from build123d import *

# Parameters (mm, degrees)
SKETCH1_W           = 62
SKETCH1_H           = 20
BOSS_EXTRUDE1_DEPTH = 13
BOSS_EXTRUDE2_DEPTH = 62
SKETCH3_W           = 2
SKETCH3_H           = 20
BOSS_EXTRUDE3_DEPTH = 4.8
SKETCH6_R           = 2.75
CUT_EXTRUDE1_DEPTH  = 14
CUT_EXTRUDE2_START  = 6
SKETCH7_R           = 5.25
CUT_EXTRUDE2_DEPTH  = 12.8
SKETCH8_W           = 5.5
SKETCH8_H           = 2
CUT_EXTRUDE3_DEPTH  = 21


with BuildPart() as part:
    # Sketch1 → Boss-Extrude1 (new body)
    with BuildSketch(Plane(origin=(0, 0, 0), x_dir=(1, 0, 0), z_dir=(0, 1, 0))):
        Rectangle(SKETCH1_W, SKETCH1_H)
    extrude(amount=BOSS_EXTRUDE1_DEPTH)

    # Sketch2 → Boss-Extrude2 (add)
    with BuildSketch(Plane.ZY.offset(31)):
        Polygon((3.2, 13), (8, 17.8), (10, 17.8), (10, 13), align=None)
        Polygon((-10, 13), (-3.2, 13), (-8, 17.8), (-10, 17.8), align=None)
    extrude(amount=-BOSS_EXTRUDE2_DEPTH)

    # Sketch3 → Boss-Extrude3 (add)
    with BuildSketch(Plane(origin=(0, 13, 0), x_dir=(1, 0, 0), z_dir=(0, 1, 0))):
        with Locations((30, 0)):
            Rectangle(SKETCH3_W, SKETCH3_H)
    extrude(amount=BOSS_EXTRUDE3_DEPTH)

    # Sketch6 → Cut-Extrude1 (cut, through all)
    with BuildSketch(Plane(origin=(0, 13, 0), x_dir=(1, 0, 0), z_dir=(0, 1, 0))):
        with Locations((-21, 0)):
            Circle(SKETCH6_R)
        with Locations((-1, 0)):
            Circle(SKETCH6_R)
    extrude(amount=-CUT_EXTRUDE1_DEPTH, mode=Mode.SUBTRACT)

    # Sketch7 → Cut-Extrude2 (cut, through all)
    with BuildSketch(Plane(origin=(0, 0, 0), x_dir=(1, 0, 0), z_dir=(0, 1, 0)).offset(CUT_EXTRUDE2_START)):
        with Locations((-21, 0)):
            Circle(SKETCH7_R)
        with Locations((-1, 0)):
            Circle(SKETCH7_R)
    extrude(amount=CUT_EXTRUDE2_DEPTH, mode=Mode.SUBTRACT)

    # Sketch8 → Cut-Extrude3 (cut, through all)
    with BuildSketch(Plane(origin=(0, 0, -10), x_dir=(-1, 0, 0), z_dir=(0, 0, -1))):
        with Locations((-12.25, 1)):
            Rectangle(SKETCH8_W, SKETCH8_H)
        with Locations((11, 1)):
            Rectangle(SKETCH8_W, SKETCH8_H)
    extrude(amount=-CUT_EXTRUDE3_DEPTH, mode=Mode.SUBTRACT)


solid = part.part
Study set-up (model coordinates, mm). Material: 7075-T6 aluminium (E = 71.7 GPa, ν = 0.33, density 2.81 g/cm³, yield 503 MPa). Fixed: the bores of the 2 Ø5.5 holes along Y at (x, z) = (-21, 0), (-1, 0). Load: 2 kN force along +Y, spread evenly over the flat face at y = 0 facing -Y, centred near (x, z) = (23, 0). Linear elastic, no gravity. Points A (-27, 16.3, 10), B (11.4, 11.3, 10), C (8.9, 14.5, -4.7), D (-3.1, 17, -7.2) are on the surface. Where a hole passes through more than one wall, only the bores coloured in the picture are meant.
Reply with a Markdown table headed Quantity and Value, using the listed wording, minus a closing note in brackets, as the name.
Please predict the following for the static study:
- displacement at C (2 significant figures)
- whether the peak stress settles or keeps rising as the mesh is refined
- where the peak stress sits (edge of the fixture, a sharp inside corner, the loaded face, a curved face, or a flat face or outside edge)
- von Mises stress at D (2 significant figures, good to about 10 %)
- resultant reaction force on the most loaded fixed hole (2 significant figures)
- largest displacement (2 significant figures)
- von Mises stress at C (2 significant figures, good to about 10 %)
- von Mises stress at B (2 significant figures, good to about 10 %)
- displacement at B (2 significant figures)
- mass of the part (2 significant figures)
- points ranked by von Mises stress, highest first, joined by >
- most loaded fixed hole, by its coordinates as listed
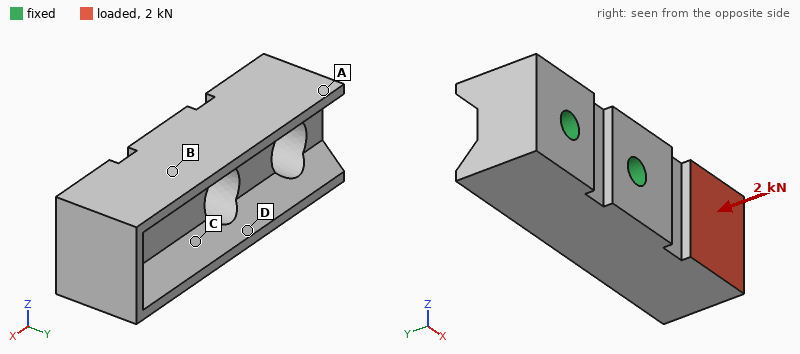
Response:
| Quantity | Value |
|---|---|
| displacement at C | 26 µm |
| whether the peak stress settles or keeps rising as the mesh is refined | keeps rising |
| where the peak stress sits | edge of the fixture |
| von Mises stress at D | 54 MPa |
| resultant reaction force on the most loaded fixed hole | 3.9 kN |
| largest displacement | 81 µm |
| von Mises stress at C | 37 MPa |
| von Mises stress at B | 25 MPa |
| displacement at B | 27 µm |
| mass of the part | 47 g |
| points ranked by von Mises stress, highest first, joined by > | D > C > B > A |
| most loaded fixed hole, by its coordinates as listed | (-1, 0) |
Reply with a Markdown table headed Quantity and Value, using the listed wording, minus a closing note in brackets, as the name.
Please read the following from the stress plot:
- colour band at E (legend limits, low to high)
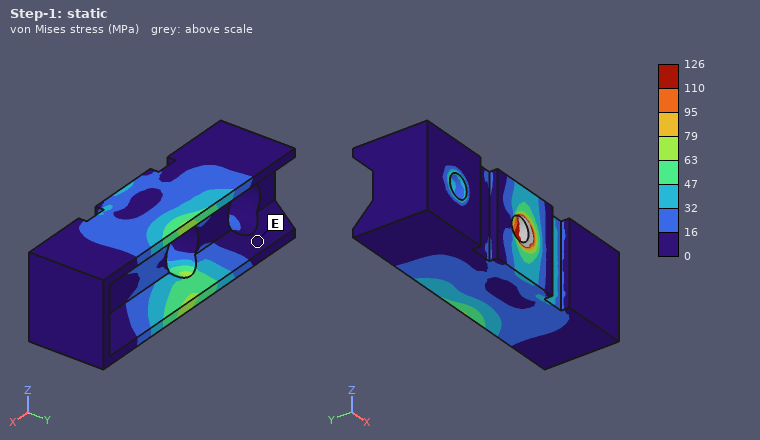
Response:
| Quantity | Value |
|---|---|
| colour band at E | 0 to 16 MPa |
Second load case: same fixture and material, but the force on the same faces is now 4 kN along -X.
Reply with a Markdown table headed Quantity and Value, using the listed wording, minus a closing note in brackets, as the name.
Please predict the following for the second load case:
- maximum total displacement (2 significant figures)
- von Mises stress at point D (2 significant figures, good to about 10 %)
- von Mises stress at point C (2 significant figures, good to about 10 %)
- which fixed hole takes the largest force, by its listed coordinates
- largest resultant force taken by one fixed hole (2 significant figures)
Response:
| Quantity | Value |
|---|---|
| maximum total displacement | 56 µm |
| von Mises stress at point D | 19 MPa |
| von Mises stress at point C | 27 MPa |
| which fixed hole takes the largest force, by its listed coordinates | (-1, 0) |
| largest resultant force taken by one fixed hole | 3.9 kN |
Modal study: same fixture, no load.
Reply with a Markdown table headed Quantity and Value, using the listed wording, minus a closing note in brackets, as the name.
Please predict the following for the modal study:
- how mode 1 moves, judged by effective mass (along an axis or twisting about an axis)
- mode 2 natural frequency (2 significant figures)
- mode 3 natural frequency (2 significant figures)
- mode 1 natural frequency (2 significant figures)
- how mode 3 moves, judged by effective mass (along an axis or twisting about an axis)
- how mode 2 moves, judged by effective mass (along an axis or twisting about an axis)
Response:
| Quantity | Value |
|---|---|
| how mode 1 moves, judged by effective mass | along Y |
| mode 2 natural frequency | 7800 Hz |
| mode 3 natural frequency | 12 kHz |
| mode 1 natural frequency | 7300 Hz |
| how mode 3 moves, judged by effective mass | twisting about X |
| how mode 2 moves, judged by effective mass | along Z |
